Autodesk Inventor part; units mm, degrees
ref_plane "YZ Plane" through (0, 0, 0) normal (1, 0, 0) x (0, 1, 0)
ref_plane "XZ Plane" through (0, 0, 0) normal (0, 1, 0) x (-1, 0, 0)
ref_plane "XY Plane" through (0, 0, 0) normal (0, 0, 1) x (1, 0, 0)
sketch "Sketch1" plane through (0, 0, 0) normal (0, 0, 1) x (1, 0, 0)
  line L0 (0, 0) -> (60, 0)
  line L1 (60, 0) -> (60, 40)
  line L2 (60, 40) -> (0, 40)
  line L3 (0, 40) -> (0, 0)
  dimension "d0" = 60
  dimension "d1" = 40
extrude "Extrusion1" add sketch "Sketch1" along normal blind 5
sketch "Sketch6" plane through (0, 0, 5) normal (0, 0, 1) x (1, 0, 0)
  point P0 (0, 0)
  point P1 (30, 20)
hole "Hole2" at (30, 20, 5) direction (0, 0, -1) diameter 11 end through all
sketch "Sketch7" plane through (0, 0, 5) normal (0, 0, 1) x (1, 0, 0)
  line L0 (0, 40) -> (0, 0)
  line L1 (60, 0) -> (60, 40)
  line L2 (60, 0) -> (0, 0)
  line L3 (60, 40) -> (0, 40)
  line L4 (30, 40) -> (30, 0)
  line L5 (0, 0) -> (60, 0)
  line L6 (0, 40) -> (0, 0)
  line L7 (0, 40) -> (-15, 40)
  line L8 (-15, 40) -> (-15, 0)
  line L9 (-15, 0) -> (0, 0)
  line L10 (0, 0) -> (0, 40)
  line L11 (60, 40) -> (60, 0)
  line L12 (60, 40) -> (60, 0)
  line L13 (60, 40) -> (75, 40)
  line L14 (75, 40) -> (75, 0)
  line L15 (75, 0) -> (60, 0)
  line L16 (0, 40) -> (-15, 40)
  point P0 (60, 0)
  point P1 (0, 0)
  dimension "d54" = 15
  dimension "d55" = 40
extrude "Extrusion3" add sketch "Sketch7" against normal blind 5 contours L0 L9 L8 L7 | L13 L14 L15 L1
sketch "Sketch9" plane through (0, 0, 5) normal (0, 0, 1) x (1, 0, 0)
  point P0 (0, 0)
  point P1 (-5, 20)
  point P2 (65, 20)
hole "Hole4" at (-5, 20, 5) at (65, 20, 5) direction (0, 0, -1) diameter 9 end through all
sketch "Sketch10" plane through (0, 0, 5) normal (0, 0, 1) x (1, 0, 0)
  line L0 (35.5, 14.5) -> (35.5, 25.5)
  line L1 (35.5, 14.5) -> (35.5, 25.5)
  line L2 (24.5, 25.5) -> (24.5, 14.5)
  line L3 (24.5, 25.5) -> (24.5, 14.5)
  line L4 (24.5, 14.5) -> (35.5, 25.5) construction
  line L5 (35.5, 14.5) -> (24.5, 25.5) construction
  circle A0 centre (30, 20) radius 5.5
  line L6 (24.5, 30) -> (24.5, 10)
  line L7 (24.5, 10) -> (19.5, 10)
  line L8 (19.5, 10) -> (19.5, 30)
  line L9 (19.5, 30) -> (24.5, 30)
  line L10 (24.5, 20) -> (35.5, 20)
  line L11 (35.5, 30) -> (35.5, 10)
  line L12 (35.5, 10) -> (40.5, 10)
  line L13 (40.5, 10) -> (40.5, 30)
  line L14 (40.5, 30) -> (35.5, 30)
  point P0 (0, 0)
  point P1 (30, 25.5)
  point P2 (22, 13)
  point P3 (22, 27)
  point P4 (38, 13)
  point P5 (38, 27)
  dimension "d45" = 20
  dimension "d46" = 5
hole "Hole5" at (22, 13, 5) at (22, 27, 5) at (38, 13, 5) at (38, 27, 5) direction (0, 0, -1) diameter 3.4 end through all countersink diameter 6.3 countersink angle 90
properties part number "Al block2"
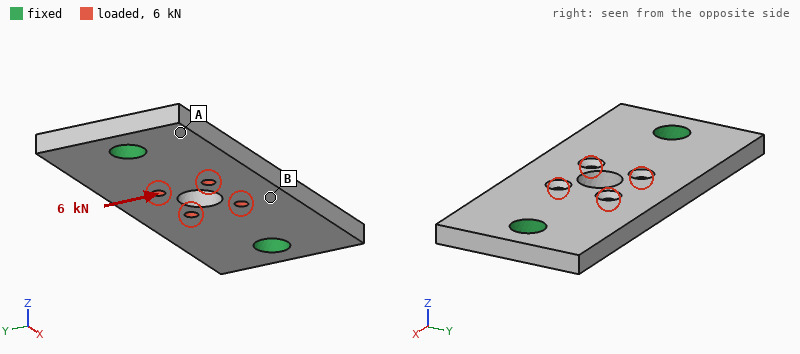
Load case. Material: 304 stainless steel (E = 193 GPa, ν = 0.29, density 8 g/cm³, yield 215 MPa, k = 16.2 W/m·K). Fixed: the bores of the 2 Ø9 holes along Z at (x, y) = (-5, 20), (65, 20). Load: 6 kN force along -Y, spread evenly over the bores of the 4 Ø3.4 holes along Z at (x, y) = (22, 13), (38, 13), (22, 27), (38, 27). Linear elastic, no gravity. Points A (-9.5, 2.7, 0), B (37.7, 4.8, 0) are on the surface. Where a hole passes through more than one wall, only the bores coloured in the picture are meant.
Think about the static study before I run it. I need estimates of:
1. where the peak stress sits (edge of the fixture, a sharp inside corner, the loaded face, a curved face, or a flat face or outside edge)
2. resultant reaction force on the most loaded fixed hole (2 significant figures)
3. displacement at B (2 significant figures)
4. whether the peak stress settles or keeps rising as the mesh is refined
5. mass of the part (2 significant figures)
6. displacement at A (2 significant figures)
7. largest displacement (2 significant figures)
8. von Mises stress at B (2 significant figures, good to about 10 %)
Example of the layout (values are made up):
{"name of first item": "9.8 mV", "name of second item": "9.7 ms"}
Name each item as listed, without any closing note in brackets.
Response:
{"where the peak stress sits": "edge of the fixture", "resultant reaction force on the most loaded fixed hole": "3.0 kN", "displacement at B": "12 µm", "whether the peak stress settles or keeps rising as the mesh is refined": "keeps rising", "mass of the part": "130 g", "displacement at A": "3.3 µm", "largest displacement": "14 µm", "von Mises stress at B": "33 MPa"}
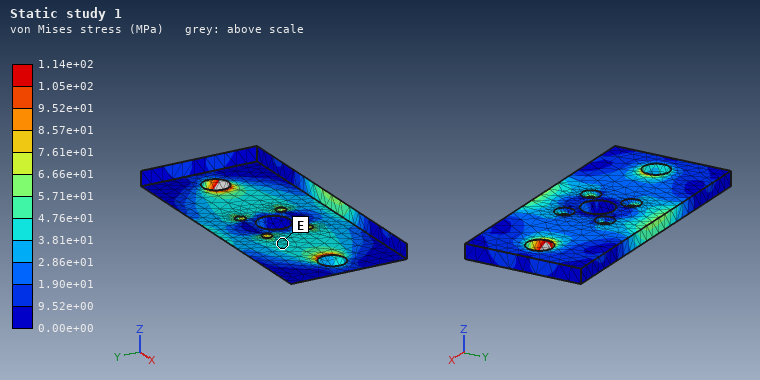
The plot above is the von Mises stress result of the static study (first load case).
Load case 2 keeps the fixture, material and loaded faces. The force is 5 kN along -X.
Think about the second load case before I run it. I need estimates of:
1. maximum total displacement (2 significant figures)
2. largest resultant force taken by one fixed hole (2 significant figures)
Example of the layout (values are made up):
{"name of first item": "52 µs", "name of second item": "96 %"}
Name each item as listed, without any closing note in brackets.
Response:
{"maximum total displacement": "3.6 µm", "largest resultant force taken by one fixed hole": "2.5 kN"}
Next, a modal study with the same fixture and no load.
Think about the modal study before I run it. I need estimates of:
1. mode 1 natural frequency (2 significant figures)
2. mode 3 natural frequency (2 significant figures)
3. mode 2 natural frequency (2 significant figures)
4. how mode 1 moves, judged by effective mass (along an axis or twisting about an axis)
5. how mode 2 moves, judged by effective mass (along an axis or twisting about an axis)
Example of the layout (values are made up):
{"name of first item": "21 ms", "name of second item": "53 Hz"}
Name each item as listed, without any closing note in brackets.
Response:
{"mode 1 natural frequency": "5100 Hz", "mode 3 natural frequency": "11 kHz", "mode 2 natural frequency": "5700 Hz", "how mode 1 moves, judged by effective mass": "along Z", "how mode 2 moves, judged by effective mass": "twisting about X"}
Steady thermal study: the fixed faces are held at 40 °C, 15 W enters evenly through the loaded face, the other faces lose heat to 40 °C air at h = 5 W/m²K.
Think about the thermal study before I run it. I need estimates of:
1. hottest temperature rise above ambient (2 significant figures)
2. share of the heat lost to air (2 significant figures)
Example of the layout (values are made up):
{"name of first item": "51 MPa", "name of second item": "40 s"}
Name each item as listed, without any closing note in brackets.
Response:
{"hottest temperature rise above ambient": "75 K", "share of the heat lost to air": "8.7 %"}
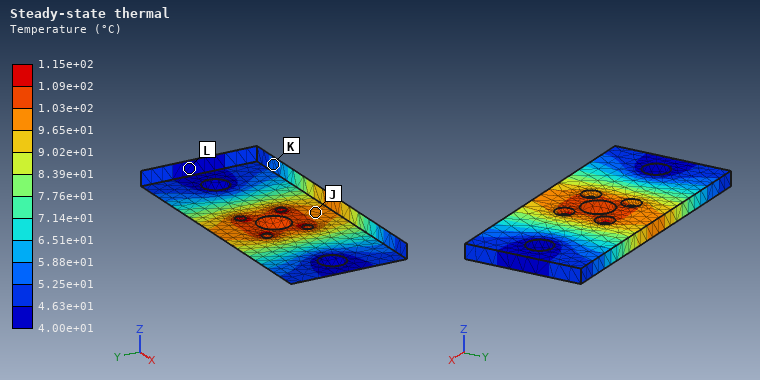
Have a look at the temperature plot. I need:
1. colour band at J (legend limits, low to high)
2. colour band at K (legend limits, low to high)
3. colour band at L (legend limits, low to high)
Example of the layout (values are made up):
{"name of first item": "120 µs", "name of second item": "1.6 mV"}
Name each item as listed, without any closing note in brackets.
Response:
{"colour band at J": "9.65e+01 to 1.03e+02 °C", "colour band at K": "5.25e+01 to 5.88e+01 °C", "colour band at L": "4.00e+01 to 4.63e+01 °C"}
